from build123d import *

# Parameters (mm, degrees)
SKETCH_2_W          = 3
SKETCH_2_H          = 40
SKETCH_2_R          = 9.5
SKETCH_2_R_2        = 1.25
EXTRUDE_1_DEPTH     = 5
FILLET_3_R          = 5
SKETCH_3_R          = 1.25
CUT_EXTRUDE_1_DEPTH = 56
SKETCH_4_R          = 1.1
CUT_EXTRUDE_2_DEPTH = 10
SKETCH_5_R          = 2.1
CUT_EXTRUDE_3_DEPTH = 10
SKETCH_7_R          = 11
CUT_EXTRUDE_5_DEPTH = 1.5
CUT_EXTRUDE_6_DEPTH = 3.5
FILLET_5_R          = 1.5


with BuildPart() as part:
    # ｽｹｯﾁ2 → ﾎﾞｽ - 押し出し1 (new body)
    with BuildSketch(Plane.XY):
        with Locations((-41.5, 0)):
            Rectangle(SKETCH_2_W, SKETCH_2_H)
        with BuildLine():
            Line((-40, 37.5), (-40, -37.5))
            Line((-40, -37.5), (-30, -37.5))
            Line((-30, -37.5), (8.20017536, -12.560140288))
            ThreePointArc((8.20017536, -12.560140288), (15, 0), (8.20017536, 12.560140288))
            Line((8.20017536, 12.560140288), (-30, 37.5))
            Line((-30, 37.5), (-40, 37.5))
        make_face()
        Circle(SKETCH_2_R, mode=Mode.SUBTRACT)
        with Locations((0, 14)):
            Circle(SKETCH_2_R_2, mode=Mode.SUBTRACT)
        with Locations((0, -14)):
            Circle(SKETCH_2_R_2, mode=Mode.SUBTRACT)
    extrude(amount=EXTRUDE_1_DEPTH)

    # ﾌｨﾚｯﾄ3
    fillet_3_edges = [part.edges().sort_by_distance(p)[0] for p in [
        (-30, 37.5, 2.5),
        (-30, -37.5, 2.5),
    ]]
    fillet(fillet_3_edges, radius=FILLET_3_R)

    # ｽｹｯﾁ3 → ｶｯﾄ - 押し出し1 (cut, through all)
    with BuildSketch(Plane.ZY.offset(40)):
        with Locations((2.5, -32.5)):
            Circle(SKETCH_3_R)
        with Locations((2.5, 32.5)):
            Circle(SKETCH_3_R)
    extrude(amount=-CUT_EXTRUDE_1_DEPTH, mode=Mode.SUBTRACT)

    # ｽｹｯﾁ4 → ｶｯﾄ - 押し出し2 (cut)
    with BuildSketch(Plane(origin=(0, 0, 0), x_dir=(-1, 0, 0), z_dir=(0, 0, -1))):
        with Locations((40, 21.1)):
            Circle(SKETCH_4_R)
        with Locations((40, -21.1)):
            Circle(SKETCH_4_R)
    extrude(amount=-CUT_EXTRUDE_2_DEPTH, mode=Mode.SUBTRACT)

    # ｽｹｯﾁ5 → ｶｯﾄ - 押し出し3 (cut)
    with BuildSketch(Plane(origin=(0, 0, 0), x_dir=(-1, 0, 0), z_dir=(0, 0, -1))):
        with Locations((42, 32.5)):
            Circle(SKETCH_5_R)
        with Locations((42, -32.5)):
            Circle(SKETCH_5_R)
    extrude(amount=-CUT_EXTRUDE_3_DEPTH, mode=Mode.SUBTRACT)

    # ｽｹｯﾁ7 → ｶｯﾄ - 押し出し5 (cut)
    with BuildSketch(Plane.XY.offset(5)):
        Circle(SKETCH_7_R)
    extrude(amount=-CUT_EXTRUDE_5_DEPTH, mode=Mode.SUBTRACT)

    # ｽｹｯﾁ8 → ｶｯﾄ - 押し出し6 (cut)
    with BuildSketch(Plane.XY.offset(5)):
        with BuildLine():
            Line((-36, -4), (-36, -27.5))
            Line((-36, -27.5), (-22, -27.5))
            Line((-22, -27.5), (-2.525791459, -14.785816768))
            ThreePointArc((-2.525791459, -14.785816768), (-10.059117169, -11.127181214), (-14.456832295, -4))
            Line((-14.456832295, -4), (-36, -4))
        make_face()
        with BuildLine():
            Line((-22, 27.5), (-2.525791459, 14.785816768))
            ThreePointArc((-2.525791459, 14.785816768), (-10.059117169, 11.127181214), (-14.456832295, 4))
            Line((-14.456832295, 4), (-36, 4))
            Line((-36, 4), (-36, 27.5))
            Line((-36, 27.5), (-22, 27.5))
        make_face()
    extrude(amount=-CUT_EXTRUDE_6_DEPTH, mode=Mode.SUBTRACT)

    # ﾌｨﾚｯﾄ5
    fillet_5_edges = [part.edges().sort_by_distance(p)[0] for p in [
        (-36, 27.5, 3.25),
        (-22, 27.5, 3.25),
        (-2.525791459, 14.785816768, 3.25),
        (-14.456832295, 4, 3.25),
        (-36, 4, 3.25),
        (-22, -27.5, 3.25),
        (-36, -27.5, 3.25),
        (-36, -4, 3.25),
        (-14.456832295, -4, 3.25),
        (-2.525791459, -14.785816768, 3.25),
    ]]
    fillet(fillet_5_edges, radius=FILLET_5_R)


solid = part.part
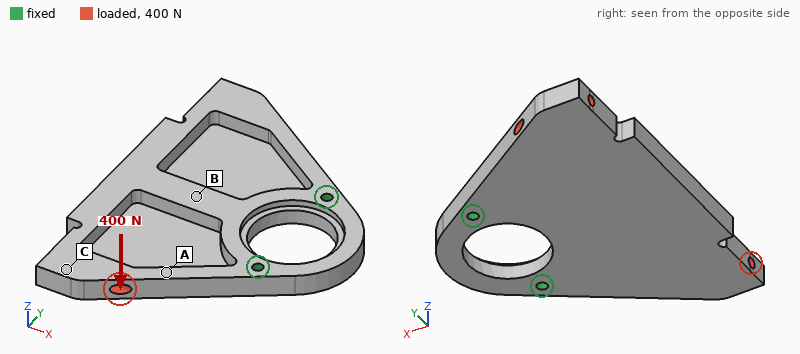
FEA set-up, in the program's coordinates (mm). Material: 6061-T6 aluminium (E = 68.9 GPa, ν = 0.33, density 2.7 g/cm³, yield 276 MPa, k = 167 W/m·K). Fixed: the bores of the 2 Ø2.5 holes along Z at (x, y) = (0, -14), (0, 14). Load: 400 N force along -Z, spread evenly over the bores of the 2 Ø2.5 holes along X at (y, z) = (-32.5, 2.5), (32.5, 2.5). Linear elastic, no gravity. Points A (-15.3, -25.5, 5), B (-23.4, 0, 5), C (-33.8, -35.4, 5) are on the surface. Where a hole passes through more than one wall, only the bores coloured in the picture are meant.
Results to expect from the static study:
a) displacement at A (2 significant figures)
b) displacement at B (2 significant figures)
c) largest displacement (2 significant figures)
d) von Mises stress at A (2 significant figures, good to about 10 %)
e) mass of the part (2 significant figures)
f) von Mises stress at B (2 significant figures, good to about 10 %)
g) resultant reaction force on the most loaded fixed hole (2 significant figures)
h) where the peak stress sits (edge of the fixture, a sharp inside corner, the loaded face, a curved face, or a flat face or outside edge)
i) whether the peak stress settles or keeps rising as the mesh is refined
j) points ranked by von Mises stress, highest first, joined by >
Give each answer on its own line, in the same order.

0.15 mm
0.20 mm
0.57 mm
86 MPa
24 g
40 MPa
220 N
edge of the fixture
keeps rising
A > B > C
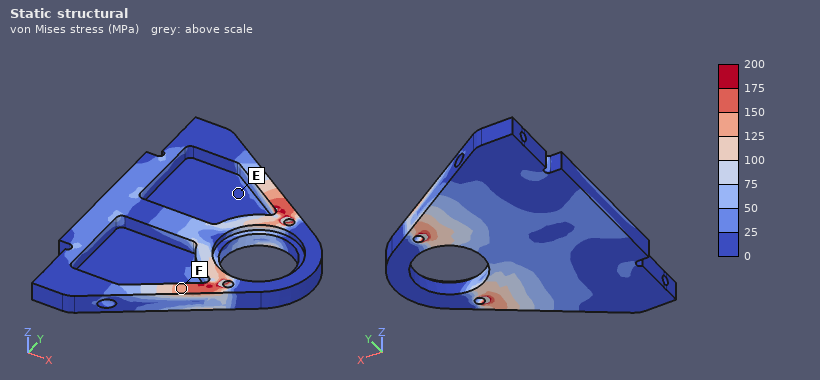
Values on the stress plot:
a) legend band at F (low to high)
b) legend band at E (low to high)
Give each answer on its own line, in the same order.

125 to 150 MPa
0 to 25 MPa
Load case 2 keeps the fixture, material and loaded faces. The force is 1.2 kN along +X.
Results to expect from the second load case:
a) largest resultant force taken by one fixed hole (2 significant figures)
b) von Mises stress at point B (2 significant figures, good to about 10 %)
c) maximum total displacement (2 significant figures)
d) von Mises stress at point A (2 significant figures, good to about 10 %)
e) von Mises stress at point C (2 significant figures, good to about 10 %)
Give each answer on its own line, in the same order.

630 N
8.1 MPa
42 µm
31 MPa
4.7 MPa
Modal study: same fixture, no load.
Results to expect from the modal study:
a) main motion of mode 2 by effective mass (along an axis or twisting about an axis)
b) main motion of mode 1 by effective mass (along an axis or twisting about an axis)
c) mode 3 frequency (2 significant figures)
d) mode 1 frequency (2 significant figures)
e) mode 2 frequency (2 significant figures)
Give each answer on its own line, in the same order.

twisting about X
along Z
4600 Hz
1300 Hz
2000 Hz
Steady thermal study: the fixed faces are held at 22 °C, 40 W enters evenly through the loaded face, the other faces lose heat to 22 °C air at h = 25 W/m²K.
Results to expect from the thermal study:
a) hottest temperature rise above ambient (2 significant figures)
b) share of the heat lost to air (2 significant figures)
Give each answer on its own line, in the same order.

72 K
17 %
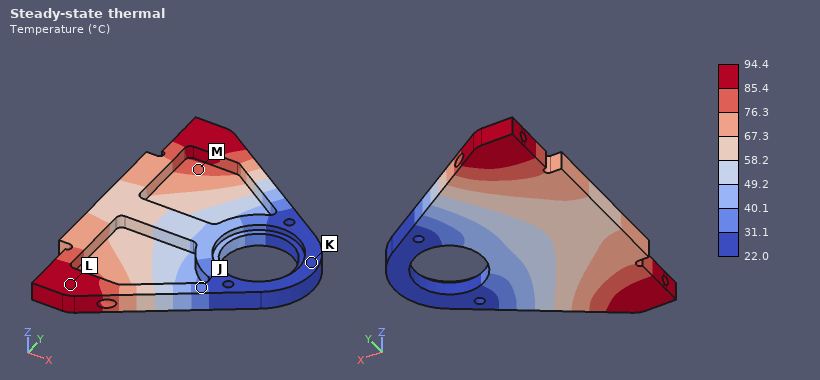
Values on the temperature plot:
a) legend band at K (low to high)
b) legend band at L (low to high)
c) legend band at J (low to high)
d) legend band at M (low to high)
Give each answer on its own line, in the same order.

22.0 to 31.1 °C
85.4 to 94.4 °C
31.1 to 40.1 °C
76.3 to 85.4 °C
